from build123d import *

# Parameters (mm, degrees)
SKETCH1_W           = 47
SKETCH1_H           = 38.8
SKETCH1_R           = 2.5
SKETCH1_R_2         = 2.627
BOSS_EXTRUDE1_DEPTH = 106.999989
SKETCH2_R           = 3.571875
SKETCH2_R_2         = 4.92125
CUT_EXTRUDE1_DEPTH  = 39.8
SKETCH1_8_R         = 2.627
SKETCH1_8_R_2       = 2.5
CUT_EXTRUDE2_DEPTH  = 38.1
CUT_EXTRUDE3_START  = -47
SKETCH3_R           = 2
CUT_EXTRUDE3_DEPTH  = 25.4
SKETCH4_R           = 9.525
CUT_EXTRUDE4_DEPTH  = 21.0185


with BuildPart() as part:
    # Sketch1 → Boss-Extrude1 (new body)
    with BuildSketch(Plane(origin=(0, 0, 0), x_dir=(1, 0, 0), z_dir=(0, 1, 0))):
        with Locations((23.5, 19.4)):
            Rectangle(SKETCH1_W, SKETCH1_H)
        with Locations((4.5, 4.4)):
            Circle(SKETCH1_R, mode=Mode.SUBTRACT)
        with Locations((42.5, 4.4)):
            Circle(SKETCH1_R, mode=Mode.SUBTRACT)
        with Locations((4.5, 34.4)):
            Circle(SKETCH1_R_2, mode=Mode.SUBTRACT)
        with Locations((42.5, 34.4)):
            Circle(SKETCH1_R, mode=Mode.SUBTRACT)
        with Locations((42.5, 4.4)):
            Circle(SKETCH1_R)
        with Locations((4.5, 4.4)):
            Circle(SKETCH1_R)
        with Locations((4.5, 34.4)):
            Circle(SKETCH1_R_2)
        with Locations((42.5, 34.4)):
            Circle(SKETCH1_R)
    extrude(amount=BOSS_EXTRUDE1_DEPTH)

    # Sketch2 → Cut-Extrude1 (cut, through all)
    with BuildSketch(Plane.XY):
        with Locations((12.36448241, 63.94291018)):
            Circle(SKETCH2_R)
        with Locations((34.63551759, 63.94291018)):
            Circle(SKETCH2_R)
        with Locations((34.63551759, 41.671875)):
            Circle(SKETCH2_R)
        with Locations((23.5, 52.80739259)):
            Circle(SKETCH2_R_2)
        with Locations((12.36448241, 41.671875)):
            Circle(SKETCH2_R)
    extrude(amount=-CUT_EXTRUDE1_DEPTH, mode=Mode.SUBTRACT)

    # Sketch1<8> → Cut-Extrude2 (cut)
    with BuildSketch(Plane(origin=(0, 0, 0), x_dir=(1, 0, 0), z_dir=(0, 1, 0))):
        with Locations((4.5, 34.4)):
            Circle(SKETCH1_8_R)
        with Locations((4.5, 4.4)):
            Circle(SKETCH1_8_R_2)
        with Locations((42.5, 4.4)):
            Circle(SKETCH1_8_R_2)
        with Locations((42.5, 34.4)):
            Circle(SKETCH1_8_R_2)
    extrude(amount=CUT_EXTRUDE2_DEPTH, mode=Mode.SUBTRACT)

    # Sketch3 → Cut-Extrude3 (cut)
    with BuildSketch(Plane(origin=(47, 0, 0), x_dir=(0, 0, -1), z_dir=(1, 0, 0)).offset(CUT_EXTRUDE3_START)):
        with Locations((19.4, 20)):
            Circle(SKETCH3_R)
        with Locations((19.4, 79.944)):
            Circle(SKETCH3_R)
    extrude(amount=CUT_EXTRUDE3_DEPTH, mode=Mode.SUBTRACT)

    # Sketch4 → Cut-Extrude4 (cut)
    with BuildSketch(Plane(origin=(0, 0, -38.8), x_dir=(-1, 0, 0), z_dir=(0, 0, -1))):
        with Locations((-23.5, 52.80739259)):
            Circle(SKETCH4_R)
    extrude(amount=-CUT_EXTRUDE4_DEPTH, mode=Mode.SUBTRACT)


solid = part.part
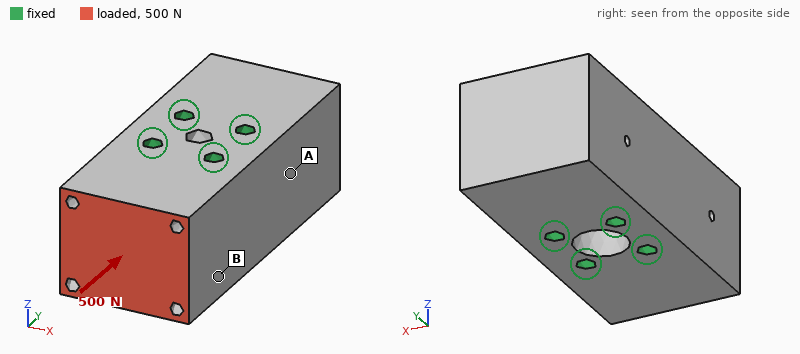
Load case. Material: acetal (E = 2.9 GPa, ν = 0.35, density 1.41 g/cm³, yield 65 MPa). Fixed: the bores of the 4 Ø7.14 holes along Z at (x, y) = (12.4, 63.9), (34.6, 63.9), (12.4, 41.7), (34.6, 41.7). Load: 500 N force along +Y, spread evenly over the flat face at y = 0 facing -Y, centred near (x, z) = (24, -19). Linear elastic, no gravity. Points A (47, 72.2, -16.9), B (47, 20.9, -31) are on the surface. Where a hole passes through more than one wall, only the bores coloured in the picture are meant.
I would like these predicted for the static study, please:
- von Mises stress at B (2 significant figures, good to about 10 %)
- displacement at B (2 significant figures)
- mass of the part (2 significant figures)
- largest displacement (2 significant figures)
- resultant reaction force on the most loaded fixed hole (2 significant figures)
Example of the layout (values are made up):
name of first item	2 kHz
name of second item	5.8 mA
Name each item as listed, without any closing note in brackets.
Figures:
von Mises stress at B	0.25 MPa
displacement at B	2.4 µm
mass of the part	250 g
largest displacement	4.5 µm
resultant reaction force on the most loaded fixed hole	230 N
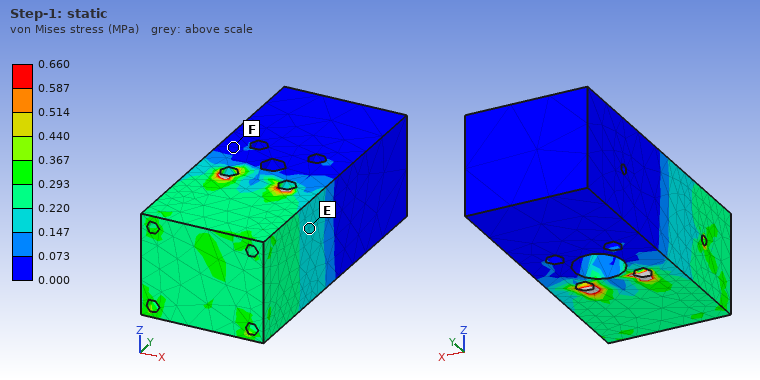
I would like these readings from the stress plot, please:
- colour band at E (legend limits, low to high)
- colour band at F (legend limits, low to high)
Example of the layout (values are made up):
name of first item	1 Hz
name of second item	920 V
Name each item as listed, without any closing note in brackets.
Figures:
colour band at E	0.147 to 0.220 MPa
colour band at F	0.000 to 0.073 MPa
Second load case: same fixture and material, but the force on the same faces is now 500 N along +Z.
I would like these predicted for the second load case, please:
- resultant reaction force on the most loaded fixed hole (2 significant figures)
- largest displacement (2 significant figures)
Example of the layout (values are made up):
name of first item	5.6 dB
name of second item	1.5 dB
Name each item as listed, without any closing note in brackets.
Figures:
resultant reaction force on the most loaded fixed hole	270 N
largest displacement	37 µm
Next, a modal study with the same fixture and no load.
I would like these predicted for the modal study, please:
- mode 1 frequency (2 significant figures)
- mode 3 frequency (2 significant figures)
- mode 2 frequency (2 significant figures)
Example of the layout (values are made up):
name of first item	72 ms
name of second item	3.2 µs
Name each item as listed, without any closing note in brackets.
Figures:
mode 1 frequency	3300 Hz
mode 3 frequency	3500 Hz
mode 2 frequency	3300 Hz
